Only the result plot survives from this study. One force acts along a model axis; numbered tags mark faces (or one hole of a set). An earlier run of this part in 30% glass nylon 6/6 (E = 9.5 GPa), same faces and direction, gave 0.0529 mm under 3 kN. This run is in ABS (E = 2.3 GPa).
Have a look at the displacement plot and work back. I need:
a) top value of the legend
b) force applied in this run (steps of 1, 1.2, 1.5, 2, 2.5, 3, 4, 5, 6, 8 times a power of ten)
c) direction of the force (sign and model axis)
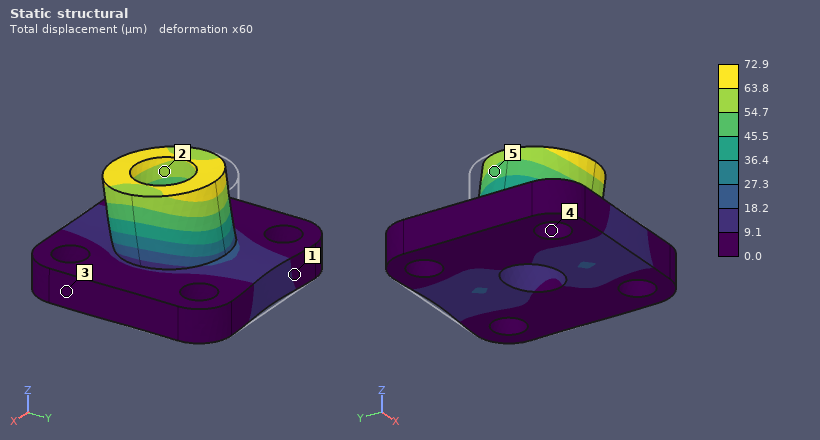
72.9 µm
1 kN
-Y
